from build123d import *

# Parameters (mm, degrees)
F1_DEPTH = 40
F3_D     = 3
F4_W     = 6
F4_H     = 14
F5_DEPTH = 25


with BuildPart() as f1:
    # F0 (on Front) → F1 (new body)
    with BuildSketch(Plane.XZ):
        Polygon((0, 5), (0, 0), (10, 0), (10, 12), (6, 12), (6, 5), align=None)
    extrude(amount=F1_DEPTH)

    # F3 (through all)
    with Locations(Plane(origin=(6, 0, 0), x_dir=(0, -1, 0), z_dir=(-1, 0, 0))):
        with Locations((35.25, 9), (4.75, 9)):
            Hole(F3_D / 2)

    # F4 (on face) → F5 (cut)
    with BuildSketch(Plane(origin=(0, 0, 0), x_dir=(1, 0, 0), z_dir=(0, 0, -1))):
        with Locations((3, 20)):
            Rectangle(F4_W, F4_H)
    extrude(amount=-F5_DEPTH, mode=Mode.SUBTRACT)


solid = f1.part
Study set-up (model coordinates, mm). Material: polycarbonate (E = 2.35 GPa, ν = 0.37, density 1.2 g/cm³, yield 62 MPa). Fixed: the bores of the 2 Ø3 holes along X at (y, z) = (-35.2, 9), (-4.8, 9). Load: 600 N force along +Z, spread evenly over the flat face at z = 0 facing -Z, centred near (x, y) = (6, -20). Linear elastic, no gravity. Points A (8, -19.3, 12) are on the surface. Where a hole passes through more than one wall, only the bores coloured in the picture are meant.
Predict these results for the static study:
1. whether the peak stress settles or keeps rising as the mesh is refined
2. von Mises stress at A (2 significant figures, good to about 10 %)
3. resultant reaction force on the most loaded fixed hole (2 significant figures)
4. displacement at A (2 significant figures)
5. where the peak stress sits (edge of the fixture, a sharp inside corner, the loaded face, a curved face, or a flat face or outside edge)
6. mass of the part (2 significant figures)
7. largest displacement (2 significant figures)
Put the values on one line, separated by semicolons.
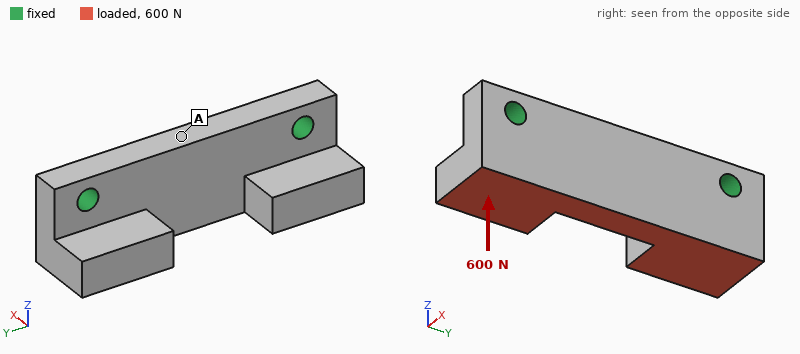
keeps rising; 4.6 MPa; 310 N; 0.098 mm; edge of the fixture; 3.2 g; 0.34 mm
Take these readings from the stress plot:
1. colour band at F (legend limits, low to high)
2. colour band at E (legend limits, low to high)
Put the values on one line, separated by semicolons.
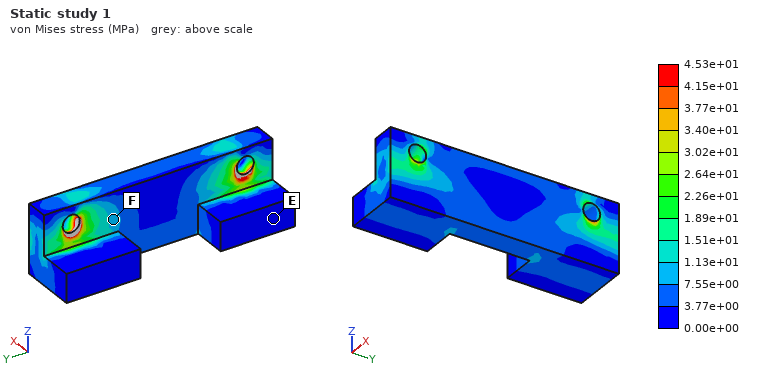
7.55e+00 to 1.13e+01 MPa; 0.00e+00 to 3.77e+00 MPa
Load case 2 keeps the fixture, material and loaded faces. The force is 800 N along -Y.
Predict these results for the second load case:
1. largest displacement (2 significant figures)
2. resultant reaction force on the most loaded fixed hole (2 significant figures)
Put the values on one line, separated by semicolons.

0.19 mm; 450 N
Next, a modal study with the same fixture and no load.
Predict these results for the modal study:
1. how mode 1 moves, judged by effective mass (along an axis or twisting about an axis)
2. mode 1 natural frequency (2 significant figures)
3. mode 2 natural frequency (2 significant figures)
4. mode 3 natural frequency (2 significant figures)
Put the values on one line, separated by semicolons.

along X; 4000 Hz; 5600 Hz; 5700 Hz
